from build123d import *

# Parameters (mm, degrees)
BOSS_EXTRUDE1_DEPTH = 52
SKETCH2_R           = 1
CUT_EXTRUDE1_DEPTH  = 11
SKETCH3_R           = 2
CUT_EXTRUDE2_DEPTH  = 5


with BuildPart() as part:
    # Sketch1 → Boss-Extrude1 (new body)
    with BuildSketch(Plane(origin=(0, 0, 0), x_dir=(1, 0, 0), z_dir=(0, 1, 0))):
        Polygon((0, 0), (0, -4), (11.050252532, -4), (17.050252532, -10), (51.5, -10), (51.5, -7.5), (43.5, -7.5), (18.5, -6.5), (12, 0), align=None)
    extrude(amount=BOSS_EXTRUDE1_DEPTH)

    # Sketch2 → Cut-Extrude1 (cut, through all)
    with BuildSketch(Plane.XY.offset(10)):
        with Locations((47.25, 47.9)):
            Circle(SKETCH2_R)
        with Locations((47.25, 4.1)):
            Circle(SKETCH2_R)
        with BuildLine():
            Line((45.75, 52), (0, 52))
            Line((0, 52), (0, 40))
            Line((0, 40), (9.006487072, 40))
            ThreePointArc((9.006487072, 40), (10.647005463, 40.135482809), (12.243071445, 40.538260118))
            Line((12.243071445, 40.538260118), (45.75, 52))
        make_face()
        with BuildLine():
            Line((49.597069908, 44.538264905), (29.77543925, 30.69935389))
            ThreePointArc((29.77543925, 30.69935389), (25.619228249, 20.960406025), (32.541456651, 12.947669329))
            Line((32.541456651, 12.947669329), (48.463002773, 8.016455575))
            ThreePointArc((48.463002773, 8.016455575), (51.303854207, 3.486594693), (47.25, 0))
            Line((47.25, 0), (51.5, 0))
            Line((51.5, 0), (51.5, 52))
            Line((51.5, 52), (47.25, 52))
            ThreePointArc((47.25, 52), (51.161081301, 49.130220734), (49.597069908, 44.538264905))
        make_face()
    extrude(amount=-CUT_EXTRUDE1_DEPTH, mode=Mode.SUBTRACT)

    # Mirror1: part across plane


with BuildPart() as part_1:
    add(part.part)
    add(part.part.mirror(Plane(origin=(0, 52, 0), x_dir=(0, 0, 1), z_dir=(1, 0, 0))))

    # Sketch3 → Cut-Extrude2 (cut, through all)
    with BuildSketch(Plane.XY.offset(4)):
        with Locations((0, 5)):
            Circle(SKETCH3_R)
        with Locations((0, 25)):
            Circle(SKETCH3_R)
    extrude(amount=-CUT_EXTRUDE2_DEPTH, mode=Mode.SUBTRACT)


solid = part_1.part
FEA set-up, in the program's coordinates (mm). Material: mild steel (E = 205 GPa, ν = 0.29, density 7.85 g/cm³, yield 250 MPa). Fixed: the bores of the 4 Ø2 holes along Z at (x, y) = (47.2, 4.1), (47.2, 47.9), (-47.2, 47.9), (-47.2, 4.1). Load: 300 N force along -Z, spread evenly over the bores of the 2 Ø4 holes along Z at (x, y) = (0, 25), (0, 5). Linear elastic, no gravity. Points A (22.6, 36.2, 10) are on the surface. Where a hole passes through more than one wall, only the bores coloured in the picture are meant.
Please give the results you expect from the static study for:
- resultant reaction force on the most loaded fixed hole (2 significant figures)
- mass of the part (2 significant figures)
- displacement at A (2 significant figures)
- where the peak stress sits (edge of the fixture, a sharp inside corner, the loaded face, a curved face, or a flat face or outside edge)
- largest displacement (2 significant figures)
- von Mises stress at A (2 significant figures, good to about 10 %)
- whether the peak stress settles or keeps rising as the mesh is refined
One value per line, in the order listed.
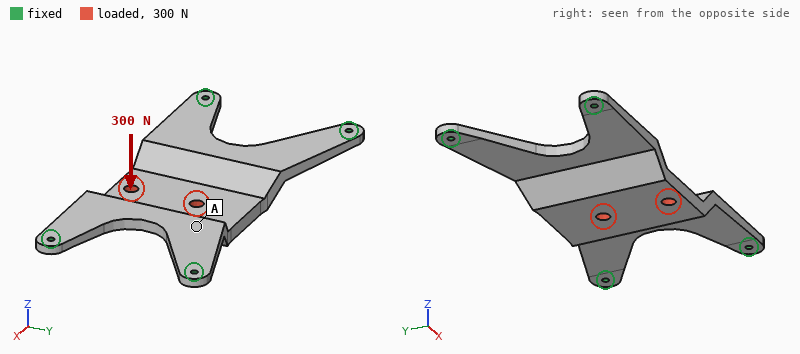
470 N
93 g
27 µm
edge of the fixture
54 µm
13 MPa
keeps rising
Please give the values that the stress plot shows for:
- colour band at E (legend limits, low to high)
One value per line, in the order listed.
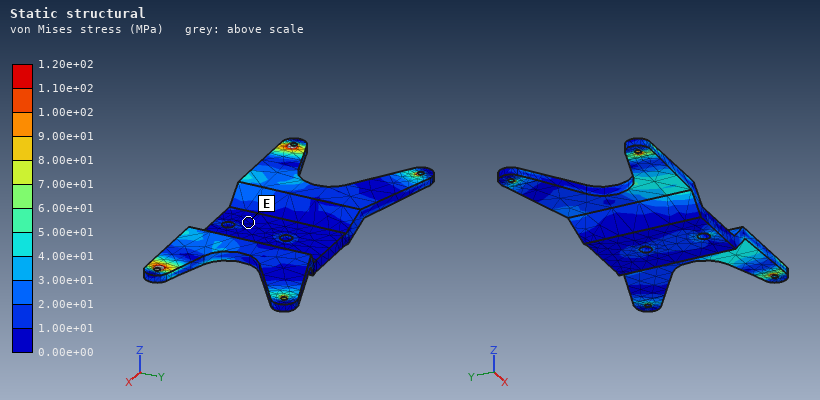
0.00e+00 to 1.00e+01 MPa
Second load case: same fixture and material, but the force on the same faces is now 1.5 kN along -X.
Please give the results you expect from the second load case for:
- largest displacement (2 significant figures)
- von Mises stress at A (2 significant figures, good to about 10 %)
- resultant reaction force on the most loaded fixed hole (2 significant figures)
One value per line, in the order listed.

17 µm
18 MPa
450 N
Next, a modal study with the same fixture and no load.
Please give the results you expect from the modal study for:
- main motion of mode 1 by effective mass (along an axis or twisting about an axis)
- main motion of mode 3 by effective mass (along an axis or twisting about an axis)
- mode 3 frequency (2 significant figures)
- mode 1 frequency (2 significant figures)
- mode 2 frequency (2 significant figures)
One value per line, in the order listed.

along Z
twisting about Y
3600 Hz
1700 Hz
2700 Hz
